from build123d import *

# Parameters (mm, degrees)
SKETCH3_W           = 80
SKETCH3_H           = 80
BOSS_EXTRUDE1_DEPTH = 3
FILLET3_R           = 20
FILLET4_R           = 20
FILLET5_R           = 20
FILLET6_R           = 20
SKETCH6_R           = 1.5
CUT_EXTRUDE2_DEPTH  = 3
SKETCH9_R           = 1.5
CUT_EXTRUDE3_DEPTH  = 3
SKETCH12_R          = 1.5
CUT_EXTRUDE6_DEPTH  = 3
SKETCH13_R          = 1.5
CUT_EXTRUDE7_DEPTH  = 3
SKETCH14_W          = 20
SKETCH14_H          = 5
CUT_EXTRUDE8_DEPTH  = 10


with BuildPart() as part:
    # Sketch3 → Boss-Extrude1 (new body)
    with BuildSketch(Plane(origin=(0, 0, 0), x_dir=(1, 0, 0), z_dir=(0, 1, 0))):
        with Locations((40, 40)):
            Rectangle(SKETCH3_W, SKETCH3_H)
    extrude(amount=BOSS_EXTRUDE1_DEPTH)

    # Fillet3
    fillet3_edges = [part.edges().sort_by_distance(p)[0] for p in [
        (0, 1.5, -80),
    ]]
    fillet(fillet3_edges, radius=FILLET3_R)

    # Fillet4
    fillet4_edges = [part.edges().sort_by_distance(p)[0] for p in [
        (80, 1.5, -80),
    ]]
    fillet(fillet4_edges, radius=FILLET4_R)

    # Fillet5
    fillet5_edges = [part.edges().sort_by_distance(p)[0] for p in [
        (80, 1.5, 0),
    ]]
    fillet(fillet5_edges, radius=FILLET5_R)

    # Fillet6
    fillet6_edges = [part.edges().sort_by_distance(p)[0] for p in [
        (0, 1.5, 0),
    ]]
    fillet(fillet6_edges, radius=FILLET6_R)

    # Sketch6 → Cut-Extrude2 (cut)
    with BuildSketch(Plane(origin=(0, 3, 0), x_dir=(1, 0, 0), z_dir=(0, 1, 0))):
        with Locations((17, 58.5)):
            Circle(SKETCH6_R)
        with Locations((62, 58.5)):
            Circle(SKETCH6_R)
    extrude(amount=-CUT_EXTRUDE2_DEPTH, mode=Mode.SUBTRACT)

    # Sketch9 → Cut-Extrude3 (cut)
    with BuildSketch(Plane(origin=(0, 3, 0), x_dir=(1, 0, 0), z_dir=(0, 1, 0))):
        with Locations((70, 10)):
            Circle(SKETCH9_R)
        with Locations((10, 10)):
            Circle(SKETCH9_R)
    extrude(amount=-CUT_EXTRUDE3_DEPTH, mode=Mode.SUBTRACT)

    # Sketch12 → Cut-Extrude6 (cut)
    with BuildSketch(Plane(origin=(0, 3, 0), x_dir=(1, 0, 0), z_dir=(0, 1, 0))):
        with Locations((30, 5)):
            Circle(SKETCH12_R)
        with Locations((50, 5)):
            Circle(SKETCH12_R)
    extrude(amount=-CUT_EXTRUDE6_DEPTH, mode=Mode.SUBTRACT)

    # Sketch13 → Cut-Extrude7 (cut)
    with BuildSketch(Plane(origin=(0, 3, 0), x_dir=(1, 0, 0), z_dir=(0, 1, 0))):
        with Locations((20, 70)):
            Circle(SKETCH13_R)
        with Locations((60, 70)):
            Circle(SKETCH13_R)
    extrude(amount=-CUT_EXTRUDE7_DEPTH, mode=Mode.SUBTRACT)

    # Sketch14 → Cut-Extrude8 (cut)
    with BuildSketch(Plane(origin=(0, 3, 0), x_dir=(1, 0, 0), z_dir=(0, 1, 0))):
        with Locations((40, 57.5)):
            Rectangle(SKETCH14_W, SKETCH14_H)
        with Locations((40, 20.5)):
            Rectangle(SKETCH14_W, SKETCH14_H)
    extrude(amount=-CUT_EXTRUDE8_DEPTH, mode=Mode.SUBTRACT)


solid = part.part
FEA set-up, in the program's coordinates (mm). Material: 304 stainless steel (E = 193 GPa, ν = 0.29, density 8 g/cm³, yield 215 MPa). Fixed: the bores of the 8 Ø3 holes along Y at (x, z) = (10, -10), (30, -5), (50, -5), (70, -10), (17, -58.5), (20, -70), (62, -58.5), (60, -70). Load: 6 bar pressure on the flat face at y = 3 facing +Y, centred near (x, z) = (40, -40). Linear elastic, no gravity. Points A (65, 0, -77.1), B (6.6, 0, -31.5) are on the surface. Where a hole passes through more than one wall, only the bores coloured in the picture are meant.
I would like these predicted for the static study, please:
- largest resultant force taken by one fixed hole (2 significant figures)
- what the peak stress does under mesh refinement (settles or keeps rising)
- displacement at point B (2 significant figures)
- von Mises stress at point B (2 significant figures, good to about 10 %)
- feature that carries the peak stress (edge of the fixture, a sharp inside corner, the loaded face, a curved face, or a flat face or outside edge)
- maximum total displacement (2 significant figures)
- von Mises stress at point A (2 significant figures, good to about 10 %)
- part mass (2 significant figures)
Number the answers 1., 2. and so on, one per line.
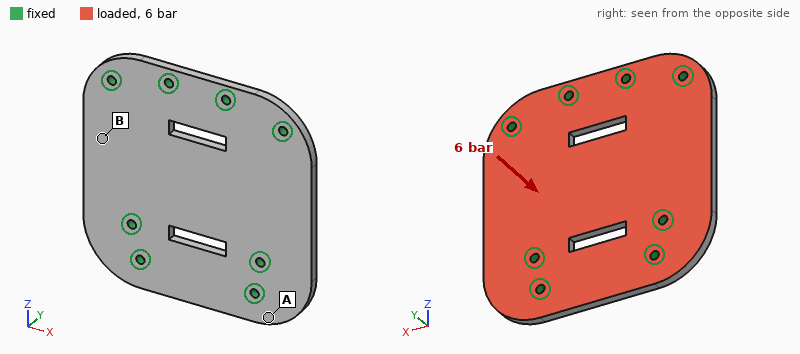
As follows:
1. 790 N
2. keeps rising
3. 28 µm
4. 45 MPa
5. edge of the fixture
6. 39 µm
7. 18 MPa
8. 140 g
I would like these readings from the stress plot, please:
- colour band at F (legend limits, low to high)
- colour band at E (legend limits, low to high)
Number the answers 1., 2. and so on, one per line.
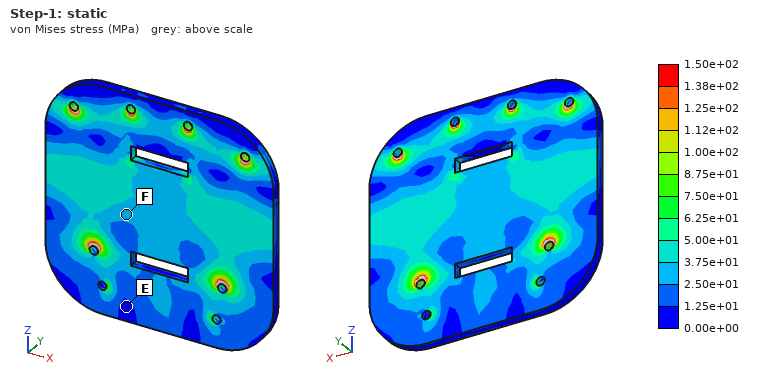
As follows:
1. 2.50e+01 to 3.75e+01 MPa
2. 0.00e+00 to 1.25e+01 MPa
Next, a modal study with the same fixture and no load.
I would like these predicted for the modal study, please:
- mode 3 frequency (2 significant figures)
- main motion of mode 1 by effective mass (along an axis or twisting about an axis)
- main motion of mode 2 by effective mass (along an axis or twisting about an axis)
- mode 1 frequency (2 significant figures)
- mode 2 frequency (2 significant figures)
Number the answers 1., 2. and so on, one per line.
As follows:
1. 5800 Hz
2. along Y
3. twisting about Z
4. 4800 Hz
5. 5500 Hz
